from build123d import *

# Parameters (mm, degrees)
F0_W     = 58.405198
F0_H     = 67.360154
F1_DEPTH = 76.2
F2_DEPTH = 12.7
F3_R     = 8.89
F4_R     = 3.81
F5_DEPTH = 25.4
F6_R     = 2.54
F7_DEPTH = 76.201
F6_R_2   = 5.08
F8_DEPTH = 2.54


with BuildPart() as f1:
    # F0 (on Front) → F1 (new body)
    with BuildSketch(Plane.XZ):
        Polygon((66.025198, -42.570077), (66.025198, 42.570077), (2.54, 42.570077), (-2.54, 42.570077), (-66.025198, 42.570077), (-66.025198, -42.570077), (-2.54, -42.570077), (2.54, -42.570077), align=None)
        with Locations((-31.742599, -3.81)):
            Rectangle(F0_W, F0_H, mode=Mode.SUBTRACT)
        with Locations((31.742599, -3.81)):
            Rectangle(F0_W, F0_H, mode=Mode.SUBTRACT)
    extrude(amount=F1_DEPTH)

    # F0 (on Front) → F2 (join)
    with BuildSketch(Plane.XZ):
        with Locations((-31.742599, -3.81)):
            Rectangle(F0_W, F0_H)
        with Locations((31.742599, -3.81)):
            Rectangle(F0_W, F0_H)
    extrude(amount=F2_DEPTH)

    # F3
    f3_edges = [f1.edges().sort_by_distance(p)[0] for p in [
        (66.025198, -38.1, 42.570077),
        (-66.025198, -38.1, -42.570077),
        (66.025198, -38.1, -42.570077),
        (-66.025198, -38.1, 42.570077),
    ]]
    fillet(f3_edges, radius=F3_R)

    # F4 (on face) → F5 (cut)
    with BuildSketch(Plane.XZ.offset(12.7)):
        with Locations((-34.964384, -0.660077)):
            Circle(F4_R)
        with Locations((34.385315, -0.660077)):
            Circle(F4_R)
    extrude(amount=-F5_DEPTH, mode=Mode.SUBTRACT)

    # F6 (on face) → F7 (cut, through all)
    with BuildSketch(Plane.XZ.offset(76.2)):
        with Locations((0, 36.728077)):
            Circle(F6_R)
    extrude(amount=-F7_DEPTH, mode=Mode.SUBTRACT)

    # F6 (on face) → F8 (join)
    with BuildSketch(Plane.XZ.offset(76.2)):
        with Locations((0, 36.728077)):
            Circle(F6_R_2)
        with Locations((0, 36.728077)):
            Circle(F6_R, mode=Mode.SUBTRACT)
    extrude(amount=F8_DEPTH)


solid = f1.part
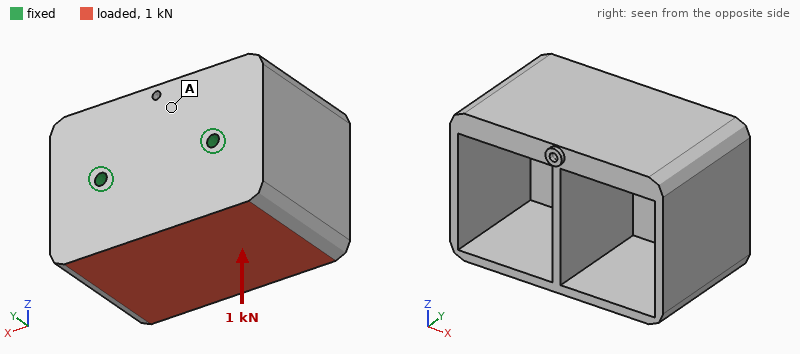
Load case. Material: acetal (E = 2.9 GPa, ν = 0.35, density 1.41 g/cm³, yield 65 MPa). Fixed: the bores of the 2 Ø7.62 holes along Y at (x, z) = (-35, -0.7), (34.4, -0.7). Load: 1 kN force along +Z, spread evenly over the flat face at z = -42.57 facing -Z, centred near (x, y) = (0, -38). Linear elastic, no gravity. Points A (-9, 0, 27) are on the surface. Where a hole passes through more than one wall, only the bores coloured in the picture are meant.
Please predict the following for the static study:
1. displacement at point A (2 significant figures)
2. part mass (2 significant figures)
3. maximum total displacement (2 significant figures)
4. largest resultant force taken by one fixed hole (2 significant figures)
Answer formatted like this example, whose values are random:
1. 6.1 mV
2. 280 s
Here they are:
1. 0.17 mm
2. 490 g
3. 0.79 mm
4. 510 N
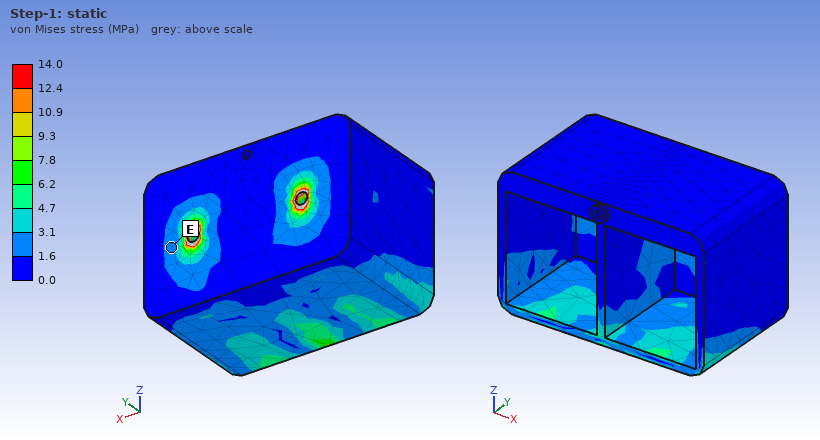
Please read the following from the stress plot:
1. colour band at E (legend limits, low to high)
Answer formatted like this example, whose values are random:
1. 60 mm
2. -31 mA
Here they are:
1. 1.6 to 3.1 MPa
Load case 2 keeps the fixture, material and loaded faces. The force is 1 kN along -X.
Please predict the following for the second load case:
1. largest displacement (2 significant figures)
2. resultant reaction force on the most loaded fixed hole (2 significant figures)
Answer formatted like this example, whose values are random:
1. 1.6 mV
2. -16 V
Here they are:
1. 0.36 mm
2. 840 N
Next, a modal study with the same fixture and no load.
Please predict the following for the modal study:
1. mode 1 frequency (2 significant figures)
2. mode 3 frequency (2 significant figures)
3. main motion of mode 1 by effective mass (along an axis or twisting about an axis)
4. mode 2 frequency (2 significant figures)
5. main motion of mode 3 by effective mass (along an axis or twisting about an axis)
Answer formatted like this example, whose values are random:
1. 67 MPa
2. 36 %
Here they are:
1. 350 Hz
2. 750 Hz
3. along Z
4. 540 Hz
5. along X
